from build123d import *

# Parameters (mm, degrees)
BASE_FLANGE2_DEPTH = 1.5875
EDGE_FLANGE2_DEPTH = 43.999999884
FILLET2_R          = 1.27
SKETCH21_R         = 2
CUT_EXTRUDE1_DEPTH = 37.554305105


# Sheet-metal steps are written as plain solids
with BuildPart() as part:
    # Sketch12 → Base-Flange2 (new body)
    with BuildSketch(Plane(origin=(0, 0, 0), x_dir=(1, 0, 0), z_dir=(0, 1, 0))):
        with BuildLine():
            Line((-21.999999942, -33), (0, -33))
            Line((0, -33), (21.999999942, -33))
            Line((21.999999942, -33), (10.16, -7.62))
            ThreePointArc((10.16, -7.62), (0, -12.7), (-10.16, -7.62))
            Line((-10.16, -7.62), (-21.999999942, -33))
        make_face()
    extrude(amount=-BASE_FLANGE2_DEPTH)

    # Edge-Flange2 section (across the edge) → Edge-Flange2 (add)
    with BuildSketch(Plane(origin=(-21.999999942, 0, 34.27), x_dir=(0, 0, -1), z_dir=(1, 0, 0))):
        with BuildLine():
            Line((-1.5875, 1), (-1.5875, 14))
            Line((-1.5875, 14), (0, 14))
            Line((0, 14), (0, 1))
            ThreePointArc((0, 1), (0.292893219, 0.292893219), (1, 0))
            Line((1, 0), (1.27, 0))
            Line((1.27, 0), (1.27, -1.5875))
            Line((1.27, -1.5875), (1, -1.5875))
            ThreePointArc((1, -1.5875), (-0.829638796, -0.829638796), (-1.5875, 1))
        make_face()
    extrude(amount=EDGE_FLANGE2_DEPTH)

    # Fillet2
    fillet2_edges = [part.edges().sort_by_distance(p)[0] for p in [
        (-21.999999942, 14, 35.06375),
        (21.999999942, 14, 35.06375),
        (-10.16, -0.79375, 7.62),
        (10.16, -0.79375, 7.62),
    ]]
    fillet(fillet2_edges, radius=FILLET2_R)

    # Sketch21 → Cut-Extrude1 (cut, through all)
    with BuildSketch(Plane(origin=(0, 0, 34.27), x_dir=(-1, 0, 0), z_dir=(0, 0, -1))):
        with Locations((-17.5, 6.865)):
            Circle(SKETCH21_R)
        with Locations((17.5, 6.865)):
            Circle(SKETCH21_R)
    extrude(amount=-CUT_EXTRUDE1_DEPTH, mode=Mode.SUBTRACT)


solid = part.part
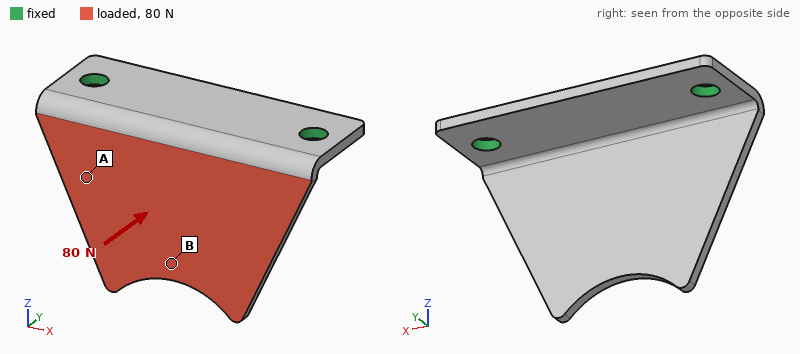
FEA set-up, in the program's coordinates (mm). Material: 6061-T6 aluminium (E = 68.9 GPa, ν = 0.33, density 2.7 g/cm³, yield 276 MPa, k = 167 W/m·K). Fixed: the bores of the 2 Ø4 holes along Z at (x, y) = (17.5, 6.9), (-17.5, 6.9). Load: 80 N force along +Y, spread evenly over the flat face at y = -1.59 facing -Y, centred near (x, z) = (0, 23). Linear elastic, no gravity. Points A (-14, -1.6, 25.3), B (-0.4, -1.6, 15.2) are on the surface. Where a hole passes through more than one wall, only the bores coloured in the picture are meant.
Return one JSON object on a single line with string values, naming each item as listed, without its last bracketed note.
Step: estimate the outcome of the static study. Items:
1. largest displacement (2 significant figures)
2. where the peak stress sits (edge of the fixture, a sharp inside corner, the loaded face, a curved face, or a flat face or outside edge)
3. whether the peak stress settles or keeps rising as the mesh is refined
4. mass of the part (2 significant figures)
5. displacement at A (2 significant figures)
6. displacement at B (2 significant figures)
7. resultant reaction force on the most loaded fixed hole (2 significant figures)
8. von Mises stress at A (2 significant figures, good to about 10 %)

{"largest displacement": "0.33 mm", "where the peak stress sits": "edge of the fixture", "whether the peak stress settles or keeps rising as the mesh is refined": "keeps rising", "mass of the part": "6.1 g", "displacement at A": "0.10 mm", "displacement at B": "0.24 mm", "resultant reaction force on the most loaded fixed hole": "41 N", "von Mises stress at A": "23 MPa"}
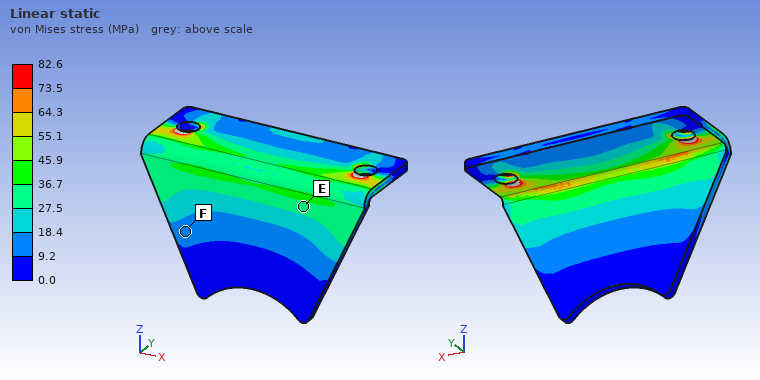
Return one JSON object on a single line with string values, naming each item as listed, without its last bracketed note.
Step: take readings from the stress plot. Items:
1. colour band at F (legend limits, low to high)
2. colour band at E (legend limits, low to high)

{"colour band at F": "9.2 to 18.4 MPa", "colour band at E": "27.5 to 36.7 MPa"}
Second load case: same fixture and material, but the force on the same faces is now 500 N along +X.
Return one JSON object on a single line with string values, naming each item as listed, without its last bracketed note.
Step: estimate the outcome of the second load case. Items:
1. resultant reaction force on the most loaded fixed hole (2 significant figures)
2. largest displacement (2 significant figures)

{"resultant reaction force on the most loaded fixed hole": "320 N", "largest displacement": "70 µm"}
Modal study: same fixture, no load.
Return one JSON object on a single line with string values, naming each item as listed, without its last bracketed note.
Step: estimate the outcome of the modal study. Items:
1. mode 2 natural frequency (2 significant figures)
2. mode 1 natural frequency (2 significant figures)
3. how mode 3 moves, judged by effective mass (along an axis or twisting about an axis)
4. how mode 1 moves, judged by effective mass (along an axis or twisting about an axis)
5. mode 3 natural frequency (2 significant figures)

{"mode 2 natural frequency": "4500 Hz", "mode 1 natural frequency": "1800 Hz", "how mode 3 moves, judged by effective mass": "along Z", "how mode 1 moves, judged by effective mass": "along Y", "mode 3 natural frequency": "7300 Hz"}
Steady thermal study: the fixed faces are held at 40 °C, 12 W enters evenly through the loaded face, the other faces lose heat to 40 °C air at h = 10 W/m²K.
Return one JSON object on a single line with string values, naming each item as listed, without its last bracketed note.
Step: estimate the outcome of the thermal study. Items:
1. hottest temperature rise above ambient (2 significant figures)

{"hottest temperature rise above ambient": "26 K"}
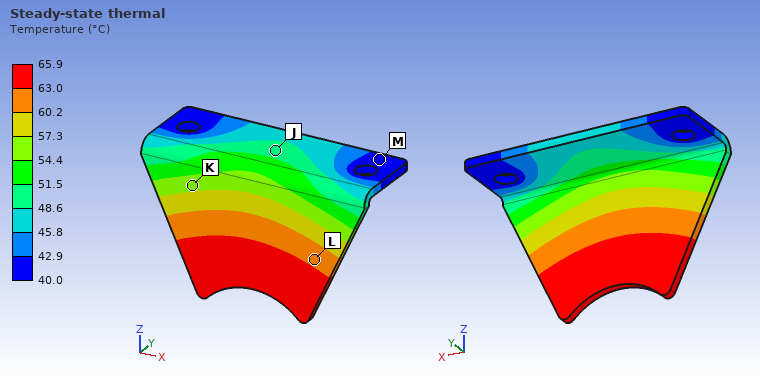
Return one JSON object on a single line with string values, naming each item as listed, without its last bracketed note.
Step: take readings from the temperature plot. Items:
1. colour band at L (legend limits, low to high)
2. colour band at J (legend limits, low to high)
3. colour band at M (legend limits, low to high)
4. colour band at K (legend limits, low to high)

{"colour band at L": "60.2 to 63.0 °C", "colour band at J": "48.6 to 51.5 °C", "colour band at M": "40.0 to 42.9 °C", "colour band at K": "54.4 to 57.3 °C"}
